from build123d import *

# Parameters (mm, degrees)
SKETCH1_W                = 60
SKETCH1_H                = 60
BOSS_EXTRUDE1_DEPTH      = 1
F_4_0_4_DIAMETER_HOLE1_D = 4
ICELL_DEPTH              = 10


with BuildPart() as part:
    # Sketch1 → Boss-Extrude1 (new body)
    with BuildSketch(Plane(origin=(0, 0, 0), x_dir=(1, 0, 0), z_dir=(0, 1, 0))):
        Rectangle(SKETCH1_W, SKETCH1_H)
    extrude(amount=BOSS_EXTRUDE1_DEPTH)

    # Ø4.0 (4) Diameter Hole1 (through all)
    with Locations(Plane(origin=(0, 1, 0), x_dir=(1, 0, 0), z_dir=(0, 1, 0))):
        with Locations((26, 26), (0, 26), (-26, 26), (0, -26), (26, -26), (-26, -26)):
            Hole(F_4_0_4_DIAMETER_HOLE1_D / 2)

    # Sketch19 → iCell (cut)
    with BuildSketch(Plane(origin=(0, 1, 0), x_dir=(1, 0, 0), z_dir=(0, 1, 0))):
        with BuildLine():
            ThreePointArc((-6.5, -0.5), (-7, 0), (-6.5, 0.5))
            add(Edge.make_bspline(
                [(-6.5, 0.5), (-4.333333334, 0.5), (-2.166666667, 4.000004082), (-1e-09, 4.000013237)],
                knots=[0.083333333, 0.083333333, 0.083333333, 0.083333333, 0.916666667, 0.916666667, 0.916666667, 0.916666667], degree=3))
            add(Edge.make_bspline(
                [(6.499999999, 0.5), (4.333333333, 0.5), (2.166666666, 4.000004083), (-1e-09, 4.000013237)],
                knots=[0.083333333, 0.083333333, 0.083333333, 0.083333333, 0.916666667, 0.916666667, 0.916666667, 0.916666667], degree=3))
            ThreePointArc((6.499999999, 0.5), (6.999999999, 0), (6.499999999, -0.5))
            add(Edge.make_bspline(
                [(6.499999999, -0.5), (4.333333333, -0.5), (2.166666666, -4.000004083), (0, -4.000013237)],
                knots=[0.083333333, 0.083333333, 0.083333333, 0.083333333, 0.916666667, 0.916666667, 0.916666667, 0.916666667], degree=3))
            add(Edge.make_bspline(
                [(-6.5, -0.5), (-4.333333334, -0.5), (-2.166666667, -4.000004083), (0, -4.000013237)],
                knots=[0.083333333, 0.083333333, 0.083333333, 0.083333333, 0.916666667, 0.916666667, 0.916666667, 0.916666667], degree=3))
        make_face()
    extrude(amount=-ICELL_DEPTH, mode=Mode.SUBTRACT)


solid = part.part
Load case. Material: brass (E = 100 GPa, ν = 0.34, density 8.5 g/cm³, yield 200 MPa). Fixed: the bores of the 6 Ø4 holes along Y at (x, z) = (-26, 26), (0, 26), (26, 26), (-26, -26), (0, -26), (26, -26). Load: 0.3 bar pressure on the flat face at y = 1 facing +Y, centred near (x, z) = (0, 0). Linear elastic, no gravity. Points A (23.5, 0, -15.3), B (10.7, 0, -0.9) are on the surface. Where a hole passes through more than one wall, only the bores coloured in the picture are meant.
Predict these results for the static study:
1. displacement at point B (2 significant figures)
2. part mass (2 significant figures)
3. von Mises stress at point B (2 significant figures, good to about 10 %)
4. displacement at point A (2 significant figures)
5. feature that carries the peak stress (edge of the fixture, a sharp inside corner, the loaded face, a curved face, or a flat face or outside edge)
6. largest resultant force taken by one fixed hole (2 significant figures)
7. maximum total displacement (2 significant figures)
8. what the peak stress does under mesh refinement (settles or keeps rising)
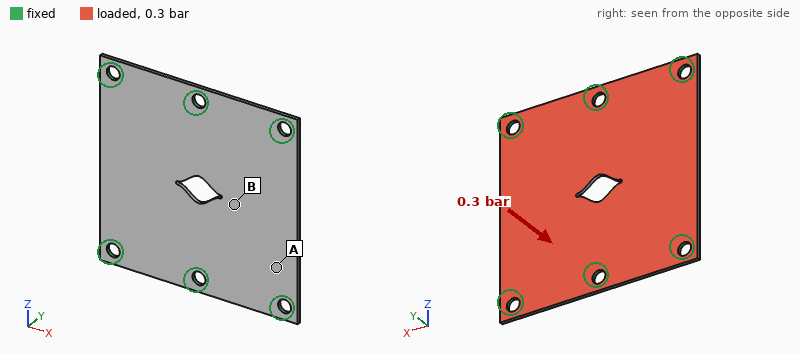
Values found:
69 µm
29 g
23 MPa
27 µm
edge of the fixture
23 N
75 µm
keeps rising
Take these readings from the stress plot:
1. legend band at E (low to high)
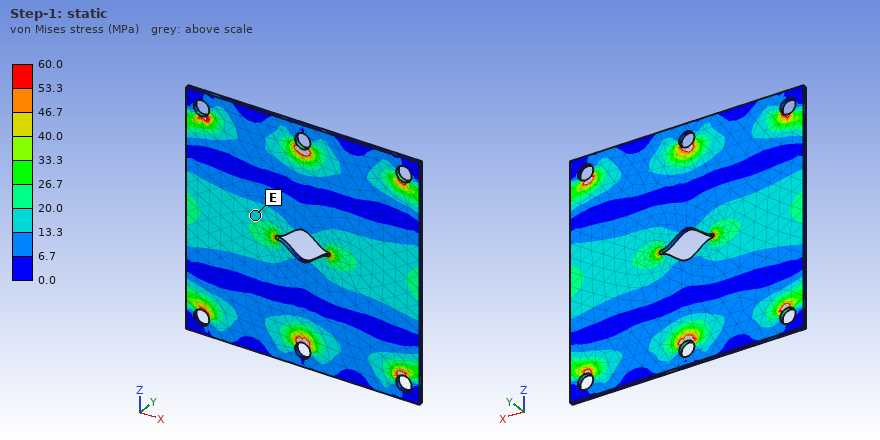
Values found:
13.3 to 20.0 MPa
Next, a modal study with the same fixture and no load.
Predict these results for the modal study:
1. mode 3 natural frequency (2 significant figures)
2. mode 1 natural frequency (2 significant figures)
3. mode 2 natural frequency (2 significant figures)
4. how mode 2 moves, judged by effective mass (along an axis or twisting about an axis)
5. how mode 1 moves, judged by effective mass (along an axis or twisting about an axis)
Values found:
2400 Hz
1300 Hz
1600 Hz
twisting about Z
along Y
